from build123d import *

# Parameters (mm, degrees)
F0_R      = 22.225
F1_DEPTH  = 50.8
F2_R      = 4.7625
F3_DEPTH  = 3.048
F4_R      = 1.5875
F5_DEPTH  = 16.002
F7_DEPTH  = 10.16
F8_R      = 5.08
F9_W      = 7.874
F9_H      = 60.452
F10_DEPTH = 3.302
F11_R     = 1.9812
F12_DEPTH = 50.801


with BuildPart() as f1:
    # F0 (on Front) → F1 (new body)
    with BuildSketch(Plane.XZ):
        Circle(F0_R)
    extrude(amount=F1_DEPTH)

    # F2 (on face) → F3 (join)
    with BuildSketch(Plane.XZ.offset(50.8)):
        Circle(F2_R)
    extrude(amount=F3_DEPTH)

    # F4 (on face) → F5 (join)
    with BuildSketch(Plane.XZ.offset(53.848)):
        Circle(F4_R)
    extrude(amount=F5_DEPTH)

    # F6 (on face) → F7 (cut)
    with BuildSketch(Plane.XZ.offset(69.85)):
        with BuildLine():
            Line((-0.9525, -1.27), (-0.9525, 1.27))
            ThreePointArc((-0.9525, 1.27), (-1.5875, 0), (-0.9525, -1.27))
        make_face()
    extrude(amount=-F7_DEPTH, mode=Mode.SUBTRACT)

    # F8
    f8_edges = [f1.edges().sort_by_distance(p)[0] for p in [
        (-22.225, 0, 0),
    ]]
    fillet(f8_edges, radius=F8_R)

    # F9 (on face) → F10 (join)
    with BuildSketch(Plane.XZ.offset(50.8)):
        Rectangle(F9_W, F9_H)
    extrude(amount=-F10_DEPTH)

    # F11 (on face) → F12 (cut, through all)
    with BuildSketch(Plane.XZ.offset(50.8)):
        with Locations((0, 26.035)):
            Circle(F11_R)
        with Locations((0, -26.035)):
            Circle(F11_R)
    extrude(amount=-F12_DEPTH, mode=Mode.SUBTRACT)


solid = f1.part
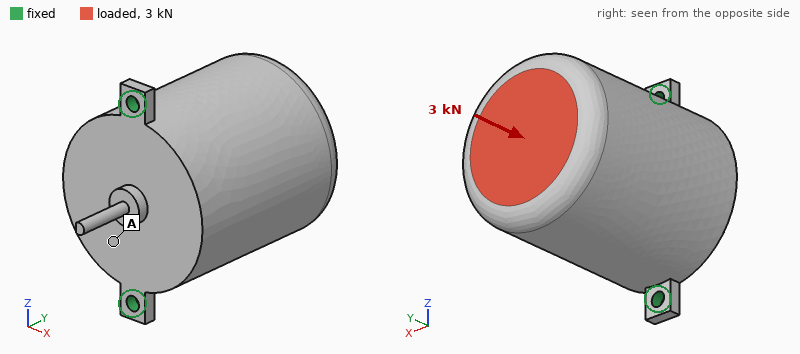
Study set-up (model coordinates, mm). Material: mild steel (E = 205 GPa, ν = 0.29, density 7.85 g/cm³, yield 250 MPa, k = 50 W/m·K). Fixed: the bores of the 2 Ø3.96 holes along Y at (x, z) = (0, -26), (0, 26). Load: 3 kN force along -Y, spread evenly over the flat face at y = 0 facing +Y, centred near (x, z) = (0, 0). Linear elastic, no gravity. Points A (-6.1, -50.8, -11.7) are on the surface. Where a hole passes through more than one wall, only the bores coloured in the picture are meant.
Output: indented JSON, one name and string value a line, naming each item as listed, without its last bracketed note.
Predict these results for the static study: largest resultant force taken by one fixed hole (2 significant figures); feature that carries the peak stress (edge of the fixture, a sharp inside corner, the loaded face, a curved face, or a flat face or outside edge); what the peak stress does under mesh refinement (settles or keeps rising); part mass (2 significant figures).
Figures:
{
  "largest resultant force taken by one fixed hole": "1.7 kN",
  "feature that carries the peak stress": "edge of the fixture",
  "what the peak stress does under mesh refinement": "keeps rising",
  "part mass": "620 g"
}
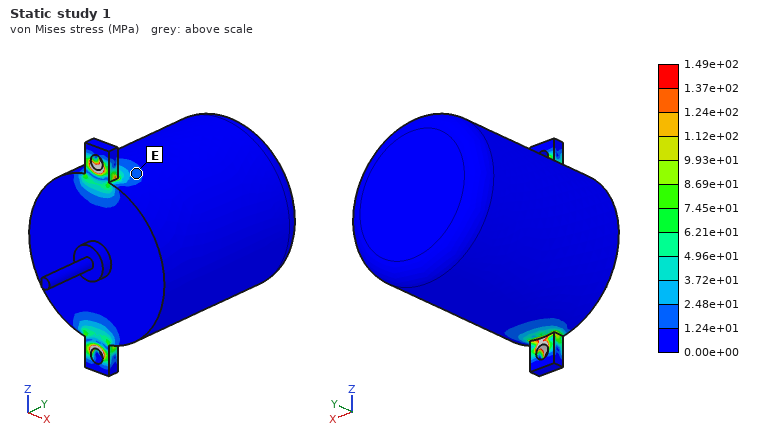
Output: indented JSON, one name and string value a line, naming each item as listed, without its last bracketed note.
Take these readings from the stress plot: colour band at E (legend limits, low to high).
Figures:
{
  "colour band at E": "1.24e+01 to 2.48e+01 MPa"
}
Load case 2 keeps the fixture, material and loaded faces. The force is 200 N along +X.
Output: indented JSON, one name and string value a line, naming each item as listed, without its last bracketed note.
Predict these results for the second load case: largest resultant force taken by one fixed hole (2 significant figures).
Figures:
{
  "largest resultant force taken by one fixed hole": "100 N"
}
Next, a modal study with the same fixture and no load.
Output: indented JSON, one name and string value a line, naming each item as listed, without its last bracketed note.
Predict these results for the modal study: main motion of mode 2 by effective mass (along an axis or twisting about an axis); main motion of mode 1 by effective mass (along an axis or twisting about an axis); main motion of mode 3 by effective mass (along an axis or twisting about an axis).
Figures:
{
  "main motion of mode 2 by effective mass": "along Z",
  "main motion of mode 1 by effective mass": "along X",
  "main motion of mode 3 by effective mass": "along Y"
}
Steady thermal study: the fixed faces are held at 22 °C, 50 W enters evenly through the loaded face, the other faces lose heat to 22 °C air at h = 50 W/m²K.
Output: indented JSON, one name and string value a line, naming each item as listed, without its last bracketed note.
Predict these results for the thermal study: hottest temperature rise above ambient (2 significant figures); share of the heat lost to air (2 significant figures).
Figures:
{
  "hottest temperature rise above ambient": "78 K",
  "share of the heat lost to air": "53 %"
}
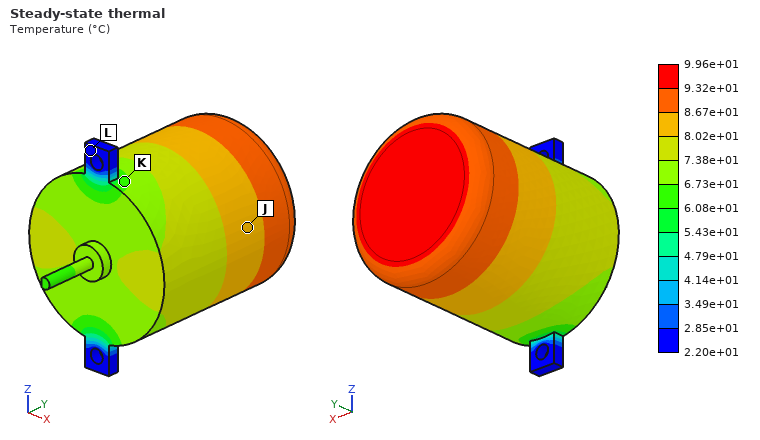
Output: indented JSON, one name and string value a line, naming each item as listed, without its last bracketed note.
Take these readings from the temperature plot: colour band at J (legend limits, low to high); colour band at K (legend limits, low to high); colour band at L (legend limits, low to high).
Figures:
{
  "colour band at J": "8.02e+01 to 8.67e+01 °C",
  "colour band at K": "6.08e+01 to 6.73e+01 °C",
  "colour band at L": "2.20e+01 to 2.85e+01 °C"
}
